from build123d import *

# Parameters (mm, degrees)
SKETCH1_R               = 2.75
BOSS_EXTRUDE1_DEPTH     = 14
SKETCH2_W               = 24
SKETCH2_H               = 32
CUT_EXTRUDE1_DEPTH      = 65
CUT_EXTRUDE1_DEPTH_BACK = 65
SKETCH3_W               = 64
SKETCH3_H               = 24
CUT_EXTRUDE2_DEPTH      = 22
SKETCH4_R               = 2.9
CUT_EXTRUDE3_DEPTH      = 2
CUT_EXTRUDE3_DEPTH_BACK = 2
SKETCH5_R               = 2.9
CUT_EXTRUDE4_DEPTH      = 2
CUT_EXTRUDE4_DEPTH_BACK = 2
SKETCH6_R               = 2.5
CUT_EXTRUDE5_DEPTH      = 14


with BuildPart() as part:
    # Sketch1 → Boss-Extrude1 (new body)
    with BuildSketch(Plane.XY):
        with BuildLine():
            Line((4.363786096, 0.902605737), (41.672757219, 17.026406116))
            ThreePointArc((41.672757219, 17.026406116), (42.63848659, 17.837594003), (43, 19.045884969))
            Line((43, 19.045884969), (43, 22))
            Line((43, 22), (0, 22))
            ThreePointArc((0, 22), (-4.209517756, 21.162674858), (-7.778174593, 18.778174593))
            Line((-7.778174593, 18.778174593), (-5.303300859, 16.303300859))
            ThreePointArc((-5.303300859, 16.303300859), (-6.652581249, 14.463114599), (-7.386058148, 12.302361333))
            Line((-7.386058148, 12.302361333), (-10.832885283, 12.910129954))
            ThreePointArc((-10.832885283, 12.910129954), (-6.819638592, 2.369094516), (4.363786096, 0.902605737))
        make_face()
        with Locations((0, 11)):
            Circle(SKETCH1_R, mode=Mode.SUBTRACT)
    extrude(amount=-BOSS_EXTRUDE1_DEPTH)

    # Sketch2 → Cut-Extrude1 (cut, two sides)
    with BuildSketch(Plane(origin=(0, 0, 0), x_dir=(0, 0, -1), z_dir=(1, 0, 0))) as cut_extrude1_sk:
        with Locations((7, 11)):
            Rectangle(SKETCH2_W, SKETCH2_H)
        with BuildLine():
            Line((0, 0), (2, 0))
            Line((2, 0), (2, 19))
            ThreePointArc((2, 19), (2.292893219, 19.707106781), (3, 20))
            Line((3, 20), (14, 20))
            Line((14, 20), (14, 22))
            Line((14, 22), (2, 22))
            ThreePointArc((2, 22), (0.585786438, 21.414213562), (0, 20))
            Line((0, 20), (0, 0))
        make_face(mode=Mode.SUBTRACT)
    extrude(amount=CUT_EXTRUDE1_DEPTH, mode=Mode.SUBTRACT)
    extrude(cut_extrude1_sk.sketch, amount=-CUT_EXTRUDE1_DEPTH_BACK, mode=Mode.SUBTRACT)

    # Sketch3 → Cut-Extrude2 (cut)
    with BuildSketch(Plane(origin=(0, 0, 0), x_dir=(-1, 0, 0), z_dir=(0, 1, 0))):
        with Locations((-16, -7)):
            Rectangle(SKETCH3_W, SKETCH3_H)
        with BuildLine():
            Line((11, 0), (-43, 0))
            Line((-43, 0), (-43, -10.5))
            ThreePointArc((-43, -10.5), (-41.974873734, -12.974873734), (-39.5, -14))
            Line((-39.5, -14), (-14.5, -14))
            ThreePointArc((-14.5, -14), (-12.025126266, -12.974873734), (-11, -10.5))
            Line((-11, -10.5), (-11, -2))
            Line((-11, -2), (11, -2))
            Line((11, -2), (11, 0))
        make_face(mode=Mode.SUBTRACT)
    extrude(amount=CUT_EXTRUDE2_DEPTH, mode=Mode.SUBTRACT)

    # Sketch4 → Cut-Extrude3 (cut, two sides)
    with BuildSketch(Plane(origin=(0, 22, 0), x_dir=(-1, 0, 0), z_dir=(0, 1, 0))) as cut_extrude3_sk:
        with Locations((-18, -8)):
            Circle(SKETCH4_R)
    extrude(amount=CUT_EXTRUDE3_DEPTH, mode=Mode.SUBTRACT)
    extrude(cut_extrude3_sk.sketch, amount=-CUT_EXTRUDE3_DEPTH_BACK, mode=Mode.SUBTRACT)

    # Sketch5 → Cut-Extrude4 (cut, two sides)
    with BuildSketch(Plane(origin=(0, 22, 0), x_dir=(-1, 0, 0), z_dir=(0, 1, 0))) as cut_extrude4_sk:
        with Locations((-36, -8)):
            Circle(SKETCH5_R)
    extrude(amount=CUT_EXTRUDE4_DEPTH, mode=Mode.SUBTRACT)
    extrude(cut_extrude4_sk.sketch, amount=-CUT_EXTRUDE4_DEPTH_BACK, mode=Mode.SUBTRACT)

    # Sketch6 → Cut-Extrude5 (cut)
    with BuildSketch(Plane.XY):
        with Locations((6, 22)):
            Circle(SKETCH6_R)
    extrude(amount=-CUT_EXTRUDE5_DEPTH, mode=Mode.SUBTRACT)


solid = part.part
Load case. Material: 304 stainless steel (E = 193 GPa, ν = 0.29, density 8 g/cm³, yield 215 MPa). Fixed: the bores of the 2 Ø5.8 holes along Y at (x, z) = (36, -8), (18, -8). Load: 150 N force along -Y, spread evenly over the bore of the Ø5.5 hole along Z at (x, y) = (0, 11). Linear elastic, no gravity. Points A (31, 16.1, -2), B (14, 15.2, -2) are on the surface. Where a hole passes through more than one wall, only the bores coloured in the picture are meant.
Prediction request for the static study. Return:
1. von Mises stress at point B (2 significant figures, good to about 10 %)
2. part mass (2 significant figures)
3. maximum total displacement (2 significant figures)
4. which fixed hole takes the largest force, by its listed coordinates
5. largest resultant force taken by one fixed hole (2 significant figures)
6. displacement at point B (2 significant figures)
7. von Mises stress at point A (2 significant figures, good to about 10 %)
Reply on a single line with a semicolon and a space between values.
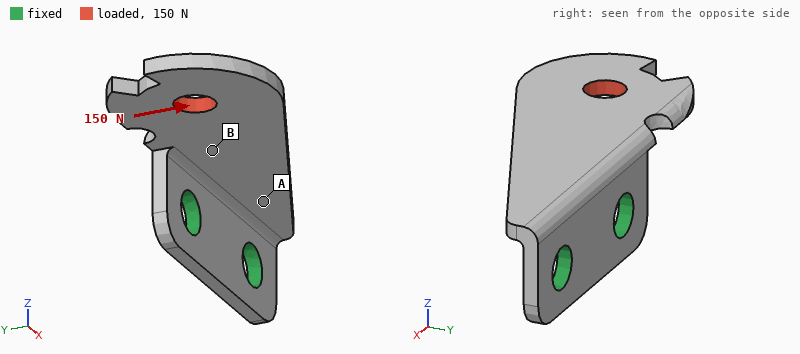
14 MPa; 17 g; 46 µm; (18, -8); 280 N; 11 µm; 34 MPa
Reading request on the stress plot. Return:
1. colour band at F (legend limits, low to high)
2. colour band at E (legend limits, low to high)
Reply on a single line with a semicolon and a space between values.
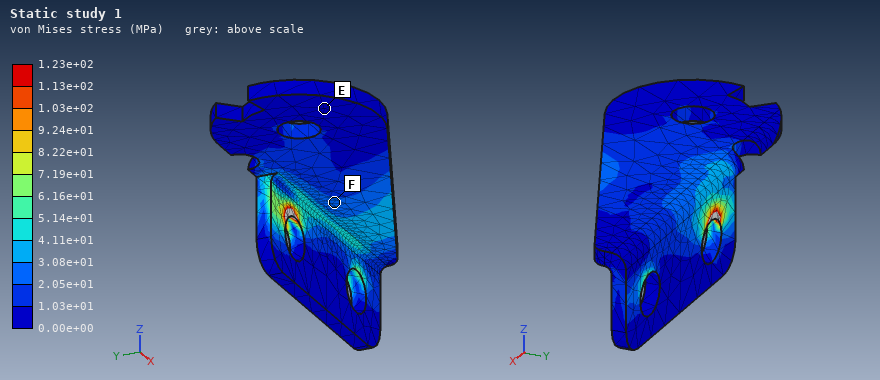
2.05e+01 to 3.08e+01 MPa; 0.00e+00 to 1.03e+01 MPa
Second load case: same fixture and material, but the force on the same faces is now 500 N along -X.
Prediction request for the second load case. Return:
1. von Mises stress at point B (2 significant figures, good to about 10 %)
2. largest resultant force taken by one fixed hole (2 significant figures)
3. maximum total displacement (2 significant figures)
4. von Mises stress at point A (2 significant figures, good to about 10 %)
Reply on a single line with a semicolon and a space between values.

24 MPa; 390 N; 41 µm; 50 MPa
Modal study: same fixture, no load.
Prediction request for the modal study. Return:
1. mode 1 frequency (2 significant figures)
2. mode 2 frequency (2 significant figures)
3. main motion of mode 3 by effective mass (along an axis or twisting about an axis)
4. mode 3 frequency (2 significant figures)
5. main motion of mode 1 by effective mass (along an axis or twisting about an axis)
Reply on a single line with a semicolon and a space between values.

1800 Hz; 4500 Hz; along Y; 5800 Hz; along Z
